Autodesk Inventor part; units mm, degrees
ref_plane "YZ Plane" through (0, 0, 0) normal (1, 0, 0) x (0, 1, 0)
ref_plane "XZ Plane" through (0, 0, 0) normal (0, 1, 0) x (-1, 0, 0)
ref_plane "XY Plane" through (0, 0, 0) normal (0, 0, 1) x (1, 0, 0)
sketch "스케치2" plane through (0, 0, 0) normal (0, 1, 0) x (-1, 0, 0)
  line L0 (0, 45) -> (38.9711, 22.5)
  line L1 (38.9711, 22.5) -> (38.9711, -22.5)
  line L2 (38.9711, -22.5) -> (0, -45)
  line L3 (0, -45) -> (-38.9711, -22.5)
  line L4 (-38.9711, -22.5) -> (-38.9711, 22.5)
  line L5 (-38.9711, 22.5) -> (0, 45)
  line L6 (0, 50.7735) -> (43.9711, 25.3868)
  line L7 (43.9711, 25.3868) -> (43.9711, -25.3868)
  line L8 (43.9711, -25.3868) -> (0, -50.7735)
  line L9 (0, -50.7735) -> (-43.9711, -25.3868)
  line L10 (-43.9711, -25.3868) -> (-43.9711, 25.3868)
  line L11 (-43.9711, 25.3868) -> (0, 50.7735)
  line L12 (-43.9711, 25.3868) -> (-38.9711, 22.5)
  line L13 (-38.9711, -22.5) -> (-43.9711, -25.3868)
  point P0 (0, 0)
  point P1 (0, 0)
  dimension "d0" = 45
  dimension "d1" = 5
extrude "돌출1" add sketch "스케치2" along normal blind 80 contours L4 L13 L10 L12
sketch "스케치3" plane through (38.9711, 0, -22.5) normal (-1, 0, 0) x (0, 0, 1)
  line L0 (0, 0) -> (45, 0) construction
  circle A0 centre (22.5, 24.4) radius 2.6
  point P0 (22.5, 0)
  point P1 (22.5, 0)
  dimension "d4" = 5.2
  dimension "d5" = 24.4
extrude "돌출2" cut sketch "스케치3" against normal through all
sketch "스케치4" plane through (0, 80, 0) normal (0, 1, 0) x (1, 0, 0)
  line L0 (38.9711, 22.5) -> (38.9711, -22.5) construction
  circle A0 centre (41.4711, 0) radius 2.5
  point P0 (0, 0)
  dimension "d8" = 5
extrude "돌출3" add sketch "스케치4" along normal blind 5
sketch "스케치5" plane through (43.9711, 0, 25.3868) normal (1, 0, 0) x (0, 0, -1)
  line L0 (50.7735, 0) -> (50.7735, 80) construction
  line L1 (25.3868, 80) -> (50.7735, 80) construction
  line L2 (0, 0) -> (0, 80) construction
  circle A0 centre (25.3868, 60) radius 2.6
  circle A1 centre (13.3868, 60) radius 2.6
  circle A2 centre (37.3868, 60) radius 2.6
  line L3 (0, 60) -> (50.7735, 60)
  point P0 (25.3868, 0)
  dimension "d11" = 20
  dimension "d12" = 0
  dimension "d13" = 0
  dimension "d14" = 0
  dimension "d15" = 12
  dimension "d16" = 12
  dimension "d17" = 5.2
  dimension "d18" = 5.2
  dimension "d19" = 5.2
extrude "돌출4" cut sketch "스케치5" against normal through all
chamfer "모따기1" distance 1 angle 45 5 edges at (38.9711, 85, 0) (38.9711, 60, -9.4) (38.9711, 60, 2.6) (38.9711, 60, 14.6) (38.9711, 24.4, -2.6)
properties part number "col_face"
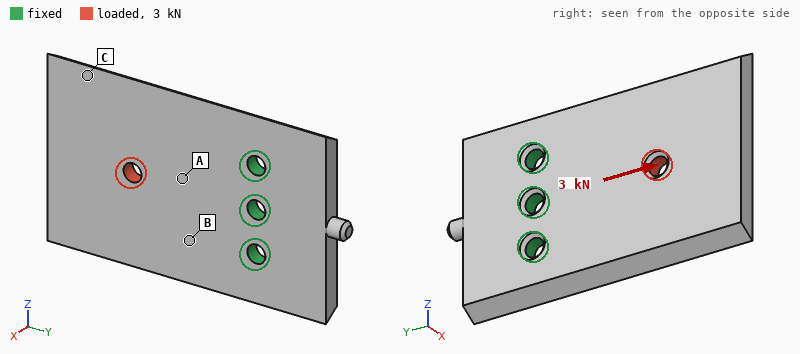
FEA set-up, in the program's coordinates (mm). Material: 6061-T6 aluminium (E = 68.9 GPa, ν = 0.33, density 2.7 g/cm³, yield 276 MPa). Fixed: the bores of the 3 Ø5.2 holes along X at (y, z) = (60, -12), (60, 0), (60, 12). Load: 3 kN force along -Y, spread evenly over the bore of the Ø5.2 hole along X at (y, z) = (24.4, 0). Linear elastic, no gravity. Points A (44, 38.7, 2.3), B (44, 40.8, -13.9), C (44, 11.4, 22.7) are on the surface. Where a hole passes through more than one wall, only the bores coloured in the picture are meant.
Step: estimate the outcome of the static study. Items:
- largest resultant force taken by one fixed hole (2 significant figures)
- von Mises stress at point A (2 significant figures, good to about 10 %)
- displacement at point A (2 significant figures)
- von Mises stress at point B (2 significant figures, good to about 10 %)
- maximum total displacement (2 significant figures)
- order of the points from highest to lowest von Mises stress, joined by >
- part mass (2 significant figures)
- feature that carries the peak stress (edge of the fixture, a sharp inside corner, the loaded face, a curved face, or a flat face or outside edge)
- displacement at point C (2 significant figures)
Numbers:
1.1 kN
27 MPa
10 µm
18 MPa
56 µm
A > B > C
51 g
the loaded face
39 µm
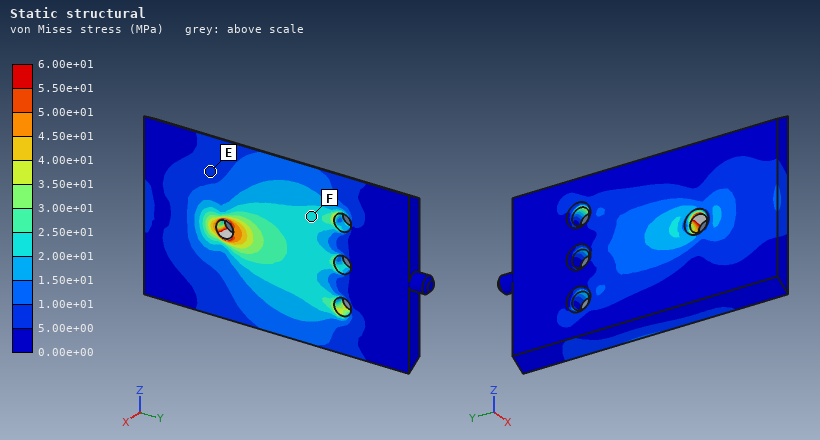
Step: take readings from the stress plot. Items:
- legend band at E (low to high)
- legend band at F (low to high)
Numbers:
5.00e+00 to 1.00e+01 MPa
2.00e+01 to 2.50e+01 MPa
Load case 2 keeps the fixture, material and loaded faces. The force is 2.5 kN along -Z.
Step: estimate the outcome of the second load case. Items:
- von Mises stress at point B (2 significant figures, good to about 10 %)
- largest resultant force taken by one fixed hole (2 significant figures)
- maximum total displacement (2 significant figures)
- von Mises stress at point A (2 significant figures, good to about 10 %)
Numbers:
27 MPa
3.3 kN
66 µm
34 MPa
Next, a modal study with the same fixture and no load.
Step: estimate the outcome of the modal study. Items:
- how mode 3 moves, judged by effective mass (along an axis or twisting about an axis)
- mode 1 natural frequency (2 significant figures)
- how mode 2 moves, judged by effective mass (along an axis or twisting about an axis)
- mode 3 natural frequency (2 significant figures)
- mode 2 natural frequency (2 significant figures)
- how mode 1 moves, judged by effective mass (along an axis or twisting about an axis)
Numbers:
along Z
1200 Hz
twisting about Y
6700 Hz
3100 Hz
along X
